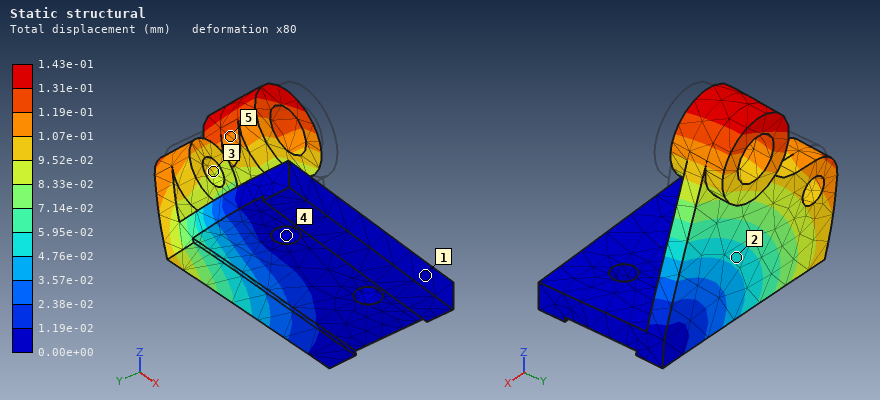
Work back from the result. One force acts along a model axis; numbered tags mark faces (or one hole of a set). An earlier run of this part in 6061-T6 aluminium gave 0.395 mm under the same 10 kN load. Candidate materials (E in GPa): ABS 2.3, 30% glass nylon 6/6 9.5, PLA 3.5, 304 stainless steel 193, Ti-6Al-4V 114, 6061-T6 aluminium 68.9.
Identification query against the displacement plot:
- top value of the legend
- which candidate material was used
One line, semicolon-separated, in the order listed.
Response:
1.43e-01 mm; 304 stainless steel
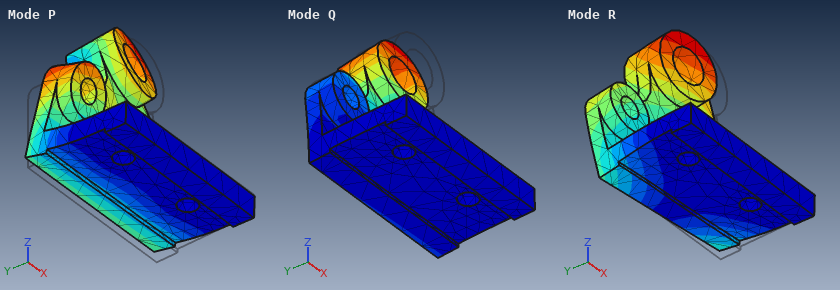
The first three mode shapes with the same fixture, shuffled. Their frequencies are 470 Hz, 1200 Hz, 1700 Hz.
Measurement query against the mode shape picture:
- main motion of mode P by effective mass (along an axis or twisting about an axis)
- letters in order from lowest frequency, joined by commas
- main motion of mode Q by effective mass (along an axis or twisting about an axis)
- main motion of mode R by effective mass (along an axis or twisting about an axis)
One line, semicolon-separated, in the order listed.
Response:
along Z; Q, R, P; along Y; along X
